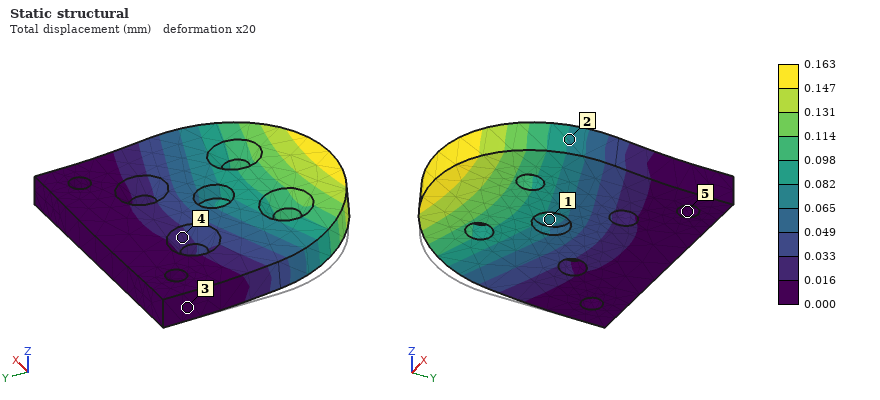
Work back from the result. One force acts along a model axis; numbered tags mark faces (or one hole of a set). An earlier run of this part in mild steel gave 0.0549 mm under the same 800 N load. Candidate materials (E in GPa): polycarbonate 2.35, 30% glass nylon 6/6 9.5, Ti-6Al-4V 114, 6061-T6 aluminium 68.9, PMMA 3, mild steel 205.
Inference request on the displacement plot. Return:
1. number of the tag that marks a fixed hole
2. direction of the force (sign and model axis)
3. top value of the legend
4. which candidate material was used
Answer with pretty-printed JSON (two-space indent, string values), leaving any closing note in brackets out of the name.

{
  "number of the tag that marks a fixed hole": "5",
  "direction of the force": "+Z",
  "top value of the legend": "0.163 mm",
  "which candidate material was used": "6061-T6 aluminium"
}
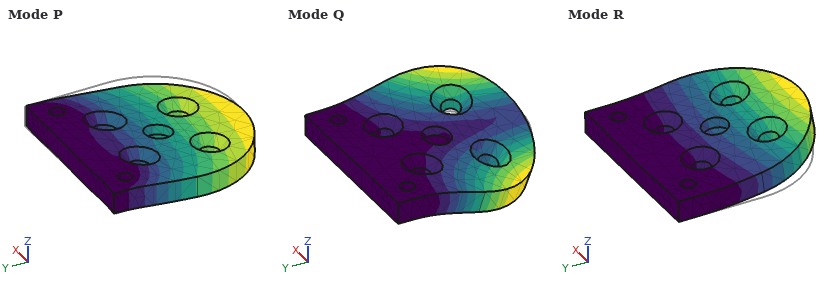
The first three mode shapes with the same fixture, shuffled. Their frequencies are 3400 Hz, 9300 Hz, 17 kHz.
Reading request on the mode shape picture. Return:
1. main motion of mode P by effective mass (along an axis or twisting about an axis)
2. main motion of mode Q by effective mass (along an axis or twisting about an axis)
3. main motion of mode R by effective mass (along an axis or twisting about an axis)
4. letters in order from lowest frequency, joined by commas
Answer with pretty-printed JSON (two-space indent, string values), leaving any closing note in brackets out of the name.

{
  "main motion of mode P by effective mass": "along X",
  "main motion of mode Q by effective mass": "twisting about Y",
  "main motion of mode R by effective mass": "along Z",
  "letters in order from lowest frequency, joined by commas": "R, Q, P"
}
